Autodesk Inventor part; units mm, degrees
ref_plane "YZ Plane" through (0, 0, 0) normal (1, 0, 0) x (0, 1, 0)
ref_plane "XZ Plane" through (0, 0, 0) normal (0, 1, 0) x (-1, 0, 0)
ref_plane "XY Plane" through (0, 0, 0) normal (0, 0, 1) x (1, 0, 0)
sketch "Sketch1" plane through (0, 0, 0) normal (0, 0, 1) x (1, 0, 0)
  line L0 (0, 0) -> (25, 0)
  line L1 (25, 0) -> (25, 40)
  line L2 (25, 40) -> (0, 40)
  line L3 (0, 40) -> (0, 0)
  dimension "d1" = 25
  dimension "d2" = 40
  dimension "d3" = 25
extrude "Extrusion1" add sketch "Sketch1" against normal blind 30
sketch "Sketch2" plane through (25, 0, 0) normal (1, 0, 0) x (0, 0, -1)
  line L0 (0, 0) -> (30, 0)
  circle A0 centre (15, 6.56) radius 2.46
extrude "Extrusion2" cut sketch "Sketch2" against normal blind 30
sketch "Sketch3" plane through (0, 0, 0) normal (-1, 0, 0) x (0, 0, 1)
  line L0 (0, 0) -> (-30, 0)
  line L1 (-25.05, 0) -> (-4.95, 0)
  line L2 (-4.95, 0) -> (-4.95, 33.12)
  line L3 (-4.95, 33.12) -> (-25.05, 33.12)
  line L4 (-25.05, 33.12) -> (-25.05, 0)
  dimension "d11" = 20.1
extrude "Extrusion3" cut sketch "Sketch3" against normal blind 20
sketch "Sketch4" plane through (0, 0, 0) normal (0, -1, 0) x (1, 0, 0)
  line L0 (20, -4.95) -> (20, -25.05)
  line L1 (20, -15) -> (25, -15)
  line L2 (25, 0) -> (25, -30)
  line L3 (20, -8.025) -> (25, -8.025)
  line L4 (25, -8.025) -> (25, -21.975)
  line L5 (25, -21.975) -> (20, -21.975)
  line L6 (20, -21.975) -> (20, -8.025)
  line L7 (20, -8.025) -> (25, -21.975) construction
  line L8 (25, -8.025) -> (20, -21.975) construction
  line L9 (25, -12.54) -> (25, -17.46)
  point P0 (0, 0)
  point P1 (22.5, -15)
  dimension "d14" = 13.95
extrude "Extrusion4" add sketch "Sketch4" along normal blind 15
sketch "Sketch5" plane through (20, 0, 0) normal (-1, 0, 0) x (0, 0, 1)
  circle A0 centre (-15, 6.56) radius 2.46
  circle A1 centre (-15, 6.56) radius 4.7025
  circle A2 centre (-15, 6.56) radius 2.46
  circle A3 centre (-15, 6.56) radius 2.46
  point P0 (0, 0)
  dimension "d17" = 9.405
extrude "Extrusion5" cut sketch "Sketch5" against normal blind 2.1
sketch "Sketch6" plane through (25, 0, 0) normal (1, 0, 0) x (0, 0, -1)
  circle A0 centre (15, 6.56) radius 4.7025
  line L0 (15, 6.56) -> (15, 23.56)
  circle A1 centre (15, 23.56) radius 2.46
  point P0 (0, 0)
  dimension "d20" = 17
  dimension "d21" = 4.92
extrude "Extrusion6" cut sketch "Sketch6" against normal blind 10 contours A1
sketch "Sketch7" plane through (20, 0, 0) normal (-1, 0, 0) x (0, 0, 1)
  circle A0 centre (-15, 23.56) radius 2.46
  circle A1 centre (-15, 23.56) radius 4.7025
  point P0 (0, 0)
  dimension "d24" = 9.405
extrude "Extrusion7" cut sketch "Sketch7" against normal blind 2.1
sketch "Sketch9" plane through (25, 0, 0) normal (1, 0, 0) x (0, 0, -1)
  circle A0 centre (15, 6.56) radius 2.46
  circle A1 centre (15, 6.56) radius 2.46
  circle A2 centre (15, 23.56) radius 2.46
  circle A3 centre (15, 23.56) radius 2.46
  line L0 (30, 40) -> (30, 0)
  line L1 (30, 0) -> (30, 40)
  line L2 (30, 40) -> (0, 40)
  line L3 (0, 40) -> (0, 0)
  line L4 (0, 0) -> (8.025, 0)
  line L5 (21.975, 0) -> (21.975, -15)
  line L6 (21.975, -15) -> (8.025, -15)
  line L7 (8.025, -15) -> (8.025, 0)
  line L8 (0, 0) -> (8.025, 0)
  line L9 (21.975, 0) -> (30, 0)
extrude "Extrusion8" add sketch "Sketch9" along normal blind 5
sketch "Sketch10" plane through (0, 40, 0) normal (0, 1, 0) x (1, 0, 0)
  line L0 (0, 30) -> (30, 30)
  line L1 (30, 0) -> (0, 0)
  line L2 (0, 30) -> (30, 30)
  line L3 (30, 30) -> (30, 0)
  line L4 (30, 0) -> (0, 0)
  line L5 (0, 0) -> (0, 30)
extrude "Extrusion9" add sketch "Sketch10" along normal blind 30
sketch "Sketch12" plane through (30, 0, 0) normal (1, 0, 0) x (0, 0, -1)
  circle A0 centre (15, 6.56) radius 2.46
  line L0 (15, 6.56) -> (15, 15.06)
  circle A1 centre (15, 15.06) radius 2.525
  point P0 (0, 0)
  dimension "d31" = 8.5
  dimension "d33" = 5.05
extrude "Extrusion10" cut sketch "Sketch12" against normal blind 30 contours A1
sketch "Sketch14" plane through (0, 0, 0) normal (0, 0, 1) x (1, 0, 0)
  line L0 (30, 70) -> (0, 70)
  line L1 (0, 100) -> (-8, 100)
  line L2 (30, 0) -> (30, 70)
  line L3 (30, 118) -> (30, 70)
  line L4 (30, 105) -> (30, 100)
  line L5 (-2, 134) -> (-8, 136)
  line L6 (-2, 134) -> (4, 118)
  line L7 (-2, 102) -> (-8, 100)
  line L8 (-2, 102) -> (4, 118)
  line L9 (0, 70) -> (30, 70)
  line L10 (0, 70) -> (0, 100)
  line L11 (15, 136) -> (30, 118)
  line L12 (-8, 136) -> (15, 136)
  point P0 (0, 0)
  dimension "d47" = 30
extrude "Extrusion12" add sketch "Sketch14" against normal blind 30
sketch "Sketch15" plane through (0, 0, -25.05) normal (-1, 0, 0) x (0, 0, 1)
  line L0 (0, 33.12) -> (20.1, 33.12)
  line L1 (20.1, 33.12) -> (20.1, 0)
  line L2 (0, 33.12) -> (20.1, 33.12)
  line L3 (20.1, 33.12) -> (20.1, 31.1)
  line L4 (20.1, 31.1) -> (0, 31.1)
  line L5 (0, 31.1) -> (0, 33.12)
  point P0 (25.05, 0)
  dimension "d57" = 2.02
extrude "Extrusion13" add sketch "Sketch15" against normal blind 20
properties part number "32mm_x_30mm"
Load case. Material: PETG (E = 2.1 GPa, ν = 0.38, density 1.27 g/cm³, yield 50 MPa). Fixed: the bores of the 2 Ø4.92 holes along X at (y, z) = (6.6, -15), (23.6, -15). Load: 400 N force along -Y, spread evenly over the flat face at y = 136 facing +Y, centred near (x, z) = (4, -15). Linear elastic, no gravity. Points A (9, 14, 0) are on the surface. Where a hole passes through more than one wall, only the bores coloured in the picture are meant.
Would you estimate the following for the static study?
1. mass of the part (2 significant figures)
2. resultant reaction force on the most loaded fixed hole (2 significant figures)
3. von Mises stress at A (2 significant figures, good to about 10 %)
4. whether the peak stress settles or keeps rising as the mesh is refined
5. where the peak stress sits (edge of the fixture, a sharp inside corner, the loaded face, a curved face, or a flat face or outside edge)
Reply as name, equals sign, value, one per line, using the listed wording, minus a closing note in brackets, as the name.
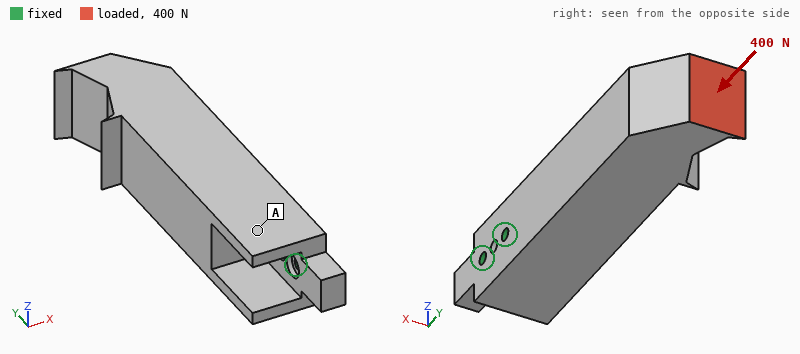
mass of the part = 140 g
resultant reaction force on the most loaded fixed hole = 410 N
von Mises stress at A = 2.0 MPa
whether the peak stress settles or keeps rising as the mesh is refined = keeps rising
where the peak stress sits = edge of the fixture
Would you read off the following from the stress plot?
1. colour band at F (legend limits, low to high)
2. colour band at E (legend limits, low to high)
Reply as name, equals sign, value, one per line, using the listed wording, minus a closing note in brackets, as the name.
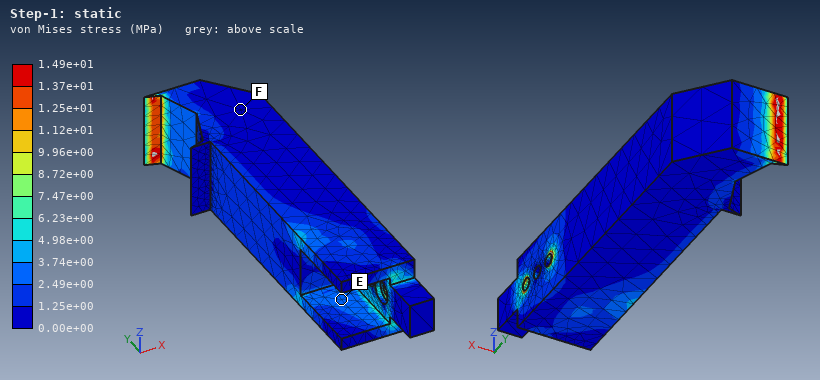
colour band at F = 0.00e+00 to 1.25e+00 MPa
colour band at E = 2.49e+00 to 3.74e+00 MPa
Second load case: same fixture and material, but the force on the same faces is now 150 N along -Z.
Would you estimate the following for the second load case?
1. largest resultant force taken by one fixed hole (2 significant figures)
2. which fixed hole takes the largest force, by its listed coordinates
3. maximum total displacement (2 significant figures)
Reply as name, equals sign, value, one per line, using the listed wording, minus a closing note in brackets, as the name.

largest resultant force taken by one fixed hole = 880 N
which fixed hole takes the largest force, by its listed coordinates = (23.6, -15)
maximum total displacement = 1.5 mm
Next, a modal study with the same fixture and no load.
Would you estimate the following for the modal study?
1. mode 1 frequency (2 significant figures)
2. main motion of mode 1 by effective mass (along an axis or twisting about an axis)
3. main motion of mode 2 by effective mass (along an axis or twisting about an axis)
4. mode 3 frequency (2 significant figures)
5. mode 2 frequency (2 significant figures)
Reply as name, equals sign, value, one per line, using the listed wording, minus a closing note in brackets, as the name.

mode 1 frequency = 240 Hz
main motion of mode 1 by effective mass = along X
main motion of mode 2 by effective mass = along Z
mode 3 frequency = 790 Hz
mode 2 frequency = 280 Hz
